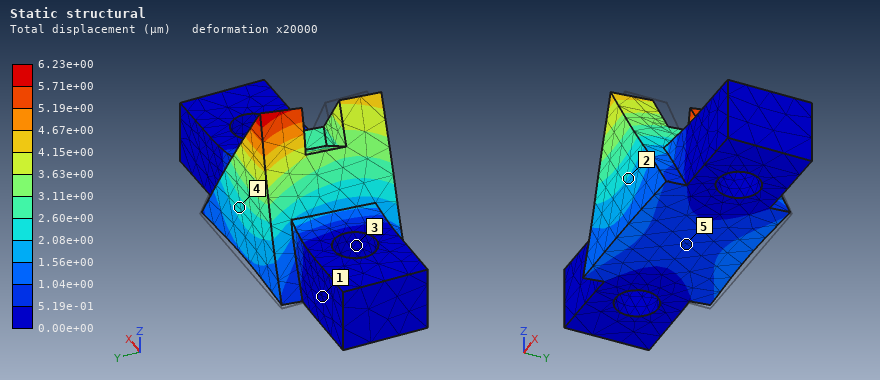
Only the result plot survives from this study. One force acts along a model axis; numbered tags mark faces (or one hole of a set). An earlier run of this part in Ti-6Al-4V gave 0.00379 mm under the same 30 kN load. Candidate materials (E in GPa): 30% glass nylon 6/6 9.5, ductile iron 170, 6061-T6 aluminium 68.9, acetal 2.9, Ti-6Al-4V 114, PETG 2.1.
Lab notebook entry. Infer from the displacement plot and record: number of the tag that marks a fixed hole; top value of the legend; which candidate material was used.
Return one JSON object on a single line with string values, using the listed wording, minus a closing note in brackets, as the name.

{"number of the tag that marks a fixed hole": "3", "top value of the legend": "6.23e+00 µm", "which candidate material was used": "6061-T6 aluminium"}
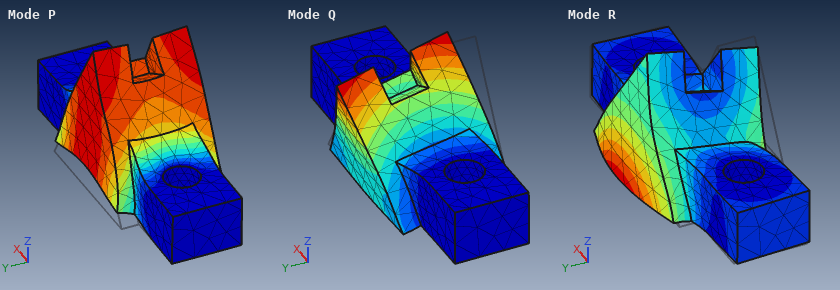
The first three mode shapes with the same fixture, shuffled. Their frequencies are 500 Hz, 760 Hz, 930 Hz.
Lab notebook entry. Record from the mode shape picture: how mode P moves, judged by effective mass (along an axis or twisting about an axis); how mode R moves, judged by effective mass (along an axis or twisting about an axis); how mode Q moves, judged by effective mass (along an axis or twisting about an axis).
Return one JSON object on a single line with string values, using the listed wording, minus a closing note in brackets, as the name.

{"how mode P moves, judged by effective mass": "along Z", "how mode R moves, judged by effective mass": "along Y", "how mode Q moves, judged by effective mass": "along Y"}
